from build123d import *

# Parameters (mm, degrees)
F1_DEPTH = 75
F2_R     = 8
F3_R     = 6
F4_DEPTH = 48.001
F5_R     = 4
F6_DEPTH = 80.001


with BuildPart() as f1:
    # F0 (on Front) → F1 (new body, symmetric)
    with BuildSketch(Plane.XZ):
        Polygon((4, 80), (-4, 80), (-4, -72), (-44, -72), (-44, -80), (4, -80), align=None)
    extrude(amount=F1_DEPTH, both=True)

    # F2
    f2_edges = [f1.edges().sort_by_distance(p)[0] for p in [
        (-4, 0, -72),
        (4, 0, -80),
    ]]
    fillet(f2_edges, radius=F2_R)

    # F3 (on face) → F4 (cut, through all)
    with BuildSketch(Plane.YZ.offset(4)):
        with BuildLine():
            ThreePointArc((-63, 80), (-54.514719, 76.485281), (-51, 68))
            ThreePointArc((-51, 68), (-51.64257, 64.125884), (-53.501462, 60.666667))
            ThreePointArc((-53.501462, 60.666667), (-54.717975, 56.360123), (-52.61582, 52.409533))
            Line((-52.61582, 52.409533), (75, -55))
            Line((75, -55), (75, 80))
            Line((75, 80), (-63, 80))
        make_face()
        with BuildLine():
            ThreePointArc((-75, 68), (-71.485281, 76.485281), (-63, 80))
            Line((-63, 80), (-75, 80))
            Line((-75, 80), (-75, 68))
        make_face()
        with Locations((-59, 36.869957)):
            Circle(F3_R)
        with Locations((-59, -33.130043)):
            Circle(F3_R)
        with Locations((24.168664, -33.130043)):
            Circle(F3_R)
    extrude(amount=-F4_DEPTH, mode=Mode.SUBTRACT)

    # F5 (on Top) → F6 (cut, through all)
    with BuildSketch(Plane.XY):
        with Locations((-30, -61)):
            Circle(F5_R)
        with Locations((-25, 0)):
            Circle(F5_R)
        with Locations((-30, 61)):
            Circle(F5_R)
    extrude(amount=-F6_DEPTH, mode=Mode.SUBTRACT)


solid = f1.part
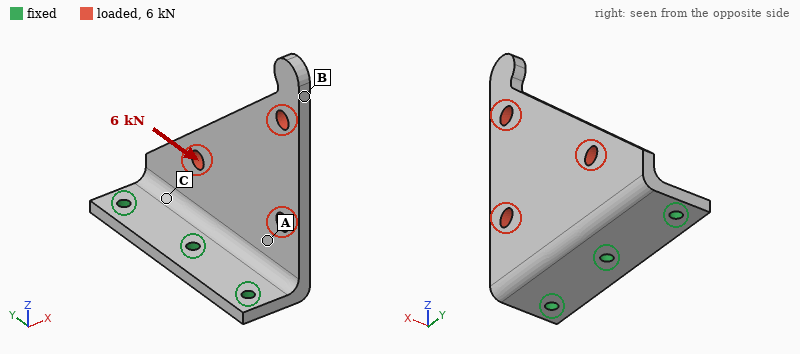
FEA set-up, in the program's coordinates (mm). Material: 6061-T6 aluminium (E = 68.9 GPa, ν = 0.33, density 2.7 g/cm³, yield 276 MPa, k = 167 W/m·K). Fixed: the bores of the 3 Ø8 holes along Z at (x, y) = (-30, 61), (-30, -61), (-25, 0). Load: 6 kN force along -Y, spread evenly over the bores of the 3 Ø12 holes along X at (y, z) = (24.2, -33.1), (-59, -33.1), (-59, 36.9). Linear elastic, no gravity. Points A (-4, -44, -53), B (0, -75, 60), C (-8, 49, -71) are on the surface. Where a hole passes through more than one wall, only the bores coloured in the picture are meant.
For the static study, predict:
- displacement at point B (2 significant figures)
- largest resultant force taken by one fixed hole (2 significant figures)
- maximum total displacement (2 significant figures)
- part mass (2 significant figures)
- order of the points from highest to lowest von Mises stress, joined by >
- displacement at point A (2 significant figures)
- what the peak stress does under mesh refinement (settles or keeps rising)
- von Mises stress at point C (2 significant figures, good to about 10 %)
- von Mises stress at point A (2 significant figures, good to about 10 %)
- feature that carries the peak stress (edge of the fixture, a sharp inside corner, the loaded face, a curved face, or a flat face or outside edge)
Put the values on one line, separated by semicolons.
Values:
0.57 mm; 3.8 kN; 0.61 mm; 410 g; C > A > B; 0.14 mm; keeps rising; 69 MPa; 36 MPa; edge of the fixture
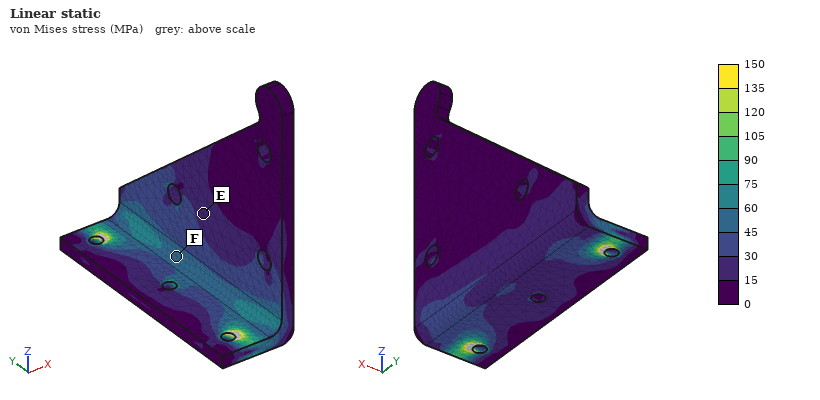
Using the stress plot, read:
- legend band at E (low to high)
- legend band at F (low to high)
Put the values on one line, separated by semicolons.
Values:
15 to 30 MPa; 45 to 60 MPa
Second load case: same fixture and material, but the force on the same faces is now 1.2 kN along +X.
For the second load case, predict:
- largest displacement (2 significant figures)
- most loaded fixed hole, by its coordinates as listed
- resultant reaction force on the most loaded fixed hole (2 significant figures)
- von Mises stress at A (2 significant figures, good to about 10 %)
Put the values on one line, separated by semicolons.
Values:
2.0 mm; (-30, -61); 690 N; 42 MPa
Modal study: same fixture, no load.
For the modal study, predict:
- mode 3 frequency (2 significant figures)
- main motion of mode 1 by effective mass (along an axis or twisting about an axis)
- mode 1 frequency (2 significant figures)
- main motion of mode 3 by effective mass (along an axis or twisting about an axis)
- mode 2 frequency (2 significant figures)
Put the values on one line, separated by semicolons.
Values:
1400 Hz; along X; 390 Hz; along Y; 1400 Hz
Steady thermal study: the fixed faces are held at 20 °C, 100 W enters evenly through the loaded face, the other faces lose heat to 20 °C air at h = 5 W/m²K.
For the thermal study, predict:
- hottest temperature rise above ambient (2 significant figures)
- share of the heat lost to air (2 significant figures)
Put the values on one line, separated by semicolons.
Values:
75 K; 5.9 %
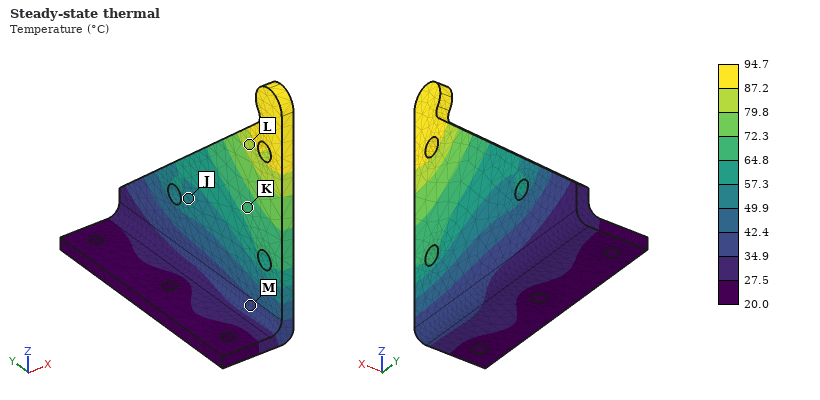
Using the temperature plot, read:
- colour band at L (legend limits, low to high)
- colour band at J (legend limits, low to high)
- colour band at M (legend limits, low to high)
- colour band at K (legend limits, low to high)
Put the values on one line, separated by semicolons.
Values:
79.8 to 87.2 °C; 49.9 to 57.3 °C; 34.9 to 42.4 °C; 64.8 to 72.3 °C
